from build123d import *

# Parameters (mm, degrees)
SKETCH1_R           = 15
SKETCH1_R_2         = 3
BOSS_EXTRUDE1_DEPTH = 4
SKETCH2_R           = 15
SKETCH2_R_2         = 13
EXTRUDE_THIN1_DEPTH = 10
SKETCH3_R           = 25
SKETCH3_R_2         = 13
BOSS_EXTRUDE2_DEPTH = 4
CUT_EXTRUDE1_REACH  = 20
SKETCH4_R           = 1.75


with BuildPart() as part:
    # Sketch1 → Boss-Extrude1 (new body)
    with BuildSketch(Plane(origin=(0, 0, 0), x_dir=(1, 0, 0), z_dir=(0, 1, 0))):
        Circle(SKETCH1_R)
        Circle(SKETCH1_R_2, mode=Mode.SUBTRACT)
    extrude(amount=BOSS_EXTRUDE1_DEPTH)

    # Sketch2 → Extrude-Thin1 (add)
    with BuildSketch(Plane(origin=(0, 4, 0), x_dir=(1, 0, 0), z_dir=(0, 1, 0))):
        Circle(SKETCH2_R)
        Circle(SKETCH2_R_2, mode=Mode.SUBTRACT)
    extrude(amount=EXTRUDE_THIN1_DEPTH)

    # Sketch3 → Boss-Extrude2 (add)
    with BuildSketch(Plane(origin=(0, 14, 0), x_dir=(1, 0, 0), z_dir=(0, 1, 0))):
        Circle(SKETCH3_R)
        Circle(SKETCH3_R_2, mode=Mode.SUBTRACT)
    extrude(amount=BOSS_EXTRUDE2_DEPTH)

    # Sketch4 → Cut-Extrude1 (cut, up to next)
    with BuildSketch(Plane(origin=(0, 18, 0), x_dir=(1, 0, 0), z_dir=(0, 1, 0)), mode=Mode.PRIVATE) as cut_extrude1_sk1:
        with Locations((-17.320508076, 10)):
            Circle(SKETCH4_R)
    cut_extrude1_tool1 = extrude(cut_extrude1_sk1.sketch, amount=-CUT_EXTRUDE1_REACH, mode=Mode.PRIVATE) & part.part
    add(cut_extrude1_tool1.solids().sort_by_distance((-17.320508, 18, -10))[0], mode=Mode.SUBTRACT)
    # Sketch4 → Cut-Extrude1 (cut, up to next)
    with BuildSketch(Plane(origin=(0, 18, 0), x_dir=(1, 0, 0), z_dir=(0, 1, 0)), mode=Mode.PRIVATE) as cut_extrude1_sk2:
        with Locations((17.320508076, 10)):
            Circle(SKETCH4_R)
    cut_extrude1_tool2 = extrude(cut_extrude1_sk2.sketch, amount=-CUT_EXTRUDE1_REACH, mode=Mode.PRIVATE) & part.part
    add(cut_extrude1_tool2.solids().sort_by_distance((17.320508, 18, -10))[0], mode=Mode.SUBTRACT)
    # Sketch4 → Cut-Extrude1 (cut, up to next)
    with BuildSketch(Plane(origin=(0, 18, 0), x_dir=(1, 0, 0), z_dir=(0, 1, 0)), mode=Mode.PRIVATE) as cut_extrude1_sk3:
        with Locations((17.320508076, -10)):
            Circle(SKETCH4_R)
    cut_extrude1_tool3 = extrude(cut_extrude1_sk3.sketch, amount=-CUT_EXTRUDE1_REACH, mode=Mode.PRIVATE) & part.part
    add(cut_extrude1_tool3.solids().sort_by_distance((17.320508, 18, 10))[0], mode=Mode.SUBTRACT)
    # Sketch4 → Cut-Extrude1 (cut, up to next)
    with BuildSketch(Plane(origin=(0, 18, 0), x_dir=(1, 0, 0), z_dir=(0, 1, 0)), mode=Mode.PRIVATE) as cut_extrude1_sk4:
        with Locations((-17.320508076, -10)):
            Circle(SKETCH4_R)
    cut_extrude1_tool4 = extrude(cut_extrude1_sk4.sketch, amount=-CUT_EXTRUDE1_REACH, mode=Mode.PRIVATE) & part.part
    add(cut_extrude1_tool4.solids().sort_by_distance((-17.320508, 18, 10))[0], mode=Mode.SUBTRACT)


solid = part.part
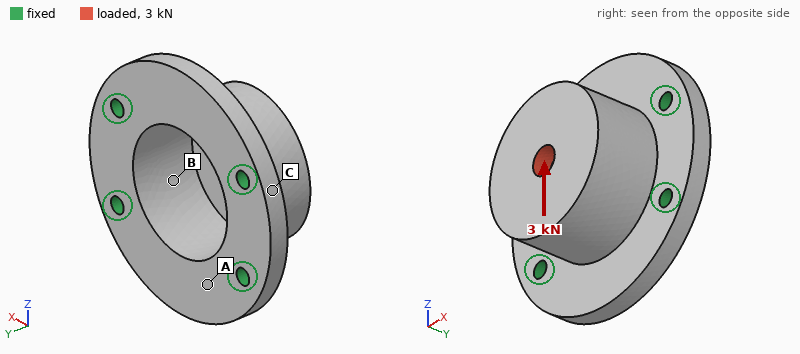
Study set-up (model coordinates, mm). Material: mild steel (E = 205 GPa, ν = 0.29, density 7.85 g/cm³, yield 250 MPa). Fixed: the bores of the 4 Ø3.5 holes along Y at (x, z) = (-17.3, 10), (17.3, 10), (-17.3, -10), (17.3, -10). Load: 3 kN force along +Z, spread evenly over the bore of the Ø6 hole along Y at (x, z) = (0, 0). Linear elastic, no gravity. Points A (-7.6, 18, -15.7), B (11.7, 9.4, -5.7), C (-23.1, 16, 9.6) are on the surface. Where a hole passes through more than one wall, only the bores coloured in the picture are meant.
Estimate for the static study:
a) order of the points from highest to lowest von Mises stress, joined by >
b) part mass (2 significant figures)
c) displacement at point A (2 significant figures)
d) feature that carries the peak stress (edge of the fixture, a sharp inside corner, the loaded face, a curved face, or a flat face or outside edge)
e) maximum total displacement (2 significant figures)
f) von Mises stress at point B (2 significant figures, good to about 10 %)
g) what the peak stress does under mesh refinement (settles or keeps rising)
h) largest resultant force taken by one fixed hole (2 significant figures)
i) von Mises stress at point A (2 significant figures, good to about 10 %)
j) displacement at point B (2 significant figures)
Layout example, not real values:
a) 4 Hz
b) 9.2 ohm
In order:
a) B > A > C
b) 79 g
c) 8.1 µm
d) edge of the fixture
e) 20 µm
f) 69 MPa
g) keeps rising
h) 1.3 kN
i) 31 MPa
j) 6.5 µm
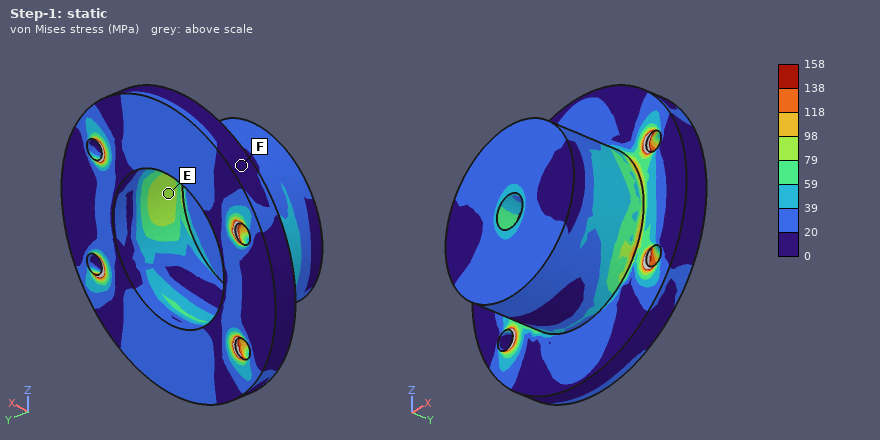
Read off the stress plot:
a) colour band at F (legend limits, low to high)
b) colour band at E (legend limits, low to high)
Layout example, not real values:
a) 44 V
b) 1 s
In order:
a) 0 to 20 MPa
b) 79 to 98 MPa
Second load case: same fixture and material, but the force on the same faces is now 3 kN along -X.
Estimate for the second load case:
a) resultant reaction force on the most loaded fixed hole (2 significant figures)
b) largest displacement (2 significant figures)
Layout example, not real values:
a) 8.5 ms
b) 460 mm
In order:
a) 1.0 kN
b) 12 µm
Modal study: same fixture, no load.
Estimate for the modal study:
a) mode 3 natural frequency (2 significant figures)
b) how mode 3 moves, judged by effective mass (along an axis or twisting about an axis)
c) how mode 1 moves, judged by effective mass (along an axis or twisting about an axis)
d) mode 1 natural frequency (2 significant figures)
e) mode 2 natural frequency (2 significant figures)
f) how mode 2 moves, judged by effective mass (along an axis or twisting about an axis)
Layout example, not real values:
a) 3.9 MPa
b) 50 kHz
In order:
a) 17 kHz
b) along X
c) along Z
d) 11 kHz
e) 15 kHz
f) along Y
